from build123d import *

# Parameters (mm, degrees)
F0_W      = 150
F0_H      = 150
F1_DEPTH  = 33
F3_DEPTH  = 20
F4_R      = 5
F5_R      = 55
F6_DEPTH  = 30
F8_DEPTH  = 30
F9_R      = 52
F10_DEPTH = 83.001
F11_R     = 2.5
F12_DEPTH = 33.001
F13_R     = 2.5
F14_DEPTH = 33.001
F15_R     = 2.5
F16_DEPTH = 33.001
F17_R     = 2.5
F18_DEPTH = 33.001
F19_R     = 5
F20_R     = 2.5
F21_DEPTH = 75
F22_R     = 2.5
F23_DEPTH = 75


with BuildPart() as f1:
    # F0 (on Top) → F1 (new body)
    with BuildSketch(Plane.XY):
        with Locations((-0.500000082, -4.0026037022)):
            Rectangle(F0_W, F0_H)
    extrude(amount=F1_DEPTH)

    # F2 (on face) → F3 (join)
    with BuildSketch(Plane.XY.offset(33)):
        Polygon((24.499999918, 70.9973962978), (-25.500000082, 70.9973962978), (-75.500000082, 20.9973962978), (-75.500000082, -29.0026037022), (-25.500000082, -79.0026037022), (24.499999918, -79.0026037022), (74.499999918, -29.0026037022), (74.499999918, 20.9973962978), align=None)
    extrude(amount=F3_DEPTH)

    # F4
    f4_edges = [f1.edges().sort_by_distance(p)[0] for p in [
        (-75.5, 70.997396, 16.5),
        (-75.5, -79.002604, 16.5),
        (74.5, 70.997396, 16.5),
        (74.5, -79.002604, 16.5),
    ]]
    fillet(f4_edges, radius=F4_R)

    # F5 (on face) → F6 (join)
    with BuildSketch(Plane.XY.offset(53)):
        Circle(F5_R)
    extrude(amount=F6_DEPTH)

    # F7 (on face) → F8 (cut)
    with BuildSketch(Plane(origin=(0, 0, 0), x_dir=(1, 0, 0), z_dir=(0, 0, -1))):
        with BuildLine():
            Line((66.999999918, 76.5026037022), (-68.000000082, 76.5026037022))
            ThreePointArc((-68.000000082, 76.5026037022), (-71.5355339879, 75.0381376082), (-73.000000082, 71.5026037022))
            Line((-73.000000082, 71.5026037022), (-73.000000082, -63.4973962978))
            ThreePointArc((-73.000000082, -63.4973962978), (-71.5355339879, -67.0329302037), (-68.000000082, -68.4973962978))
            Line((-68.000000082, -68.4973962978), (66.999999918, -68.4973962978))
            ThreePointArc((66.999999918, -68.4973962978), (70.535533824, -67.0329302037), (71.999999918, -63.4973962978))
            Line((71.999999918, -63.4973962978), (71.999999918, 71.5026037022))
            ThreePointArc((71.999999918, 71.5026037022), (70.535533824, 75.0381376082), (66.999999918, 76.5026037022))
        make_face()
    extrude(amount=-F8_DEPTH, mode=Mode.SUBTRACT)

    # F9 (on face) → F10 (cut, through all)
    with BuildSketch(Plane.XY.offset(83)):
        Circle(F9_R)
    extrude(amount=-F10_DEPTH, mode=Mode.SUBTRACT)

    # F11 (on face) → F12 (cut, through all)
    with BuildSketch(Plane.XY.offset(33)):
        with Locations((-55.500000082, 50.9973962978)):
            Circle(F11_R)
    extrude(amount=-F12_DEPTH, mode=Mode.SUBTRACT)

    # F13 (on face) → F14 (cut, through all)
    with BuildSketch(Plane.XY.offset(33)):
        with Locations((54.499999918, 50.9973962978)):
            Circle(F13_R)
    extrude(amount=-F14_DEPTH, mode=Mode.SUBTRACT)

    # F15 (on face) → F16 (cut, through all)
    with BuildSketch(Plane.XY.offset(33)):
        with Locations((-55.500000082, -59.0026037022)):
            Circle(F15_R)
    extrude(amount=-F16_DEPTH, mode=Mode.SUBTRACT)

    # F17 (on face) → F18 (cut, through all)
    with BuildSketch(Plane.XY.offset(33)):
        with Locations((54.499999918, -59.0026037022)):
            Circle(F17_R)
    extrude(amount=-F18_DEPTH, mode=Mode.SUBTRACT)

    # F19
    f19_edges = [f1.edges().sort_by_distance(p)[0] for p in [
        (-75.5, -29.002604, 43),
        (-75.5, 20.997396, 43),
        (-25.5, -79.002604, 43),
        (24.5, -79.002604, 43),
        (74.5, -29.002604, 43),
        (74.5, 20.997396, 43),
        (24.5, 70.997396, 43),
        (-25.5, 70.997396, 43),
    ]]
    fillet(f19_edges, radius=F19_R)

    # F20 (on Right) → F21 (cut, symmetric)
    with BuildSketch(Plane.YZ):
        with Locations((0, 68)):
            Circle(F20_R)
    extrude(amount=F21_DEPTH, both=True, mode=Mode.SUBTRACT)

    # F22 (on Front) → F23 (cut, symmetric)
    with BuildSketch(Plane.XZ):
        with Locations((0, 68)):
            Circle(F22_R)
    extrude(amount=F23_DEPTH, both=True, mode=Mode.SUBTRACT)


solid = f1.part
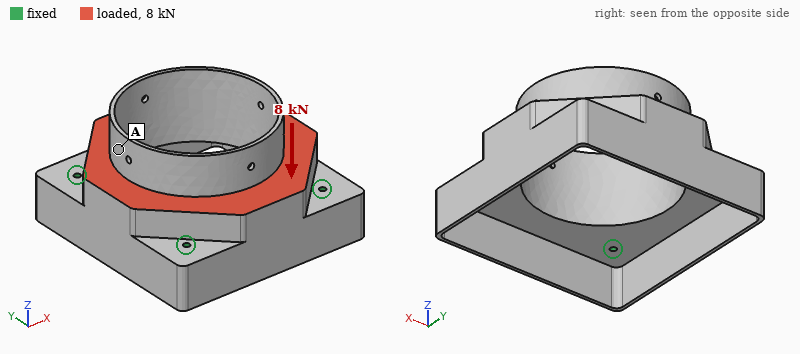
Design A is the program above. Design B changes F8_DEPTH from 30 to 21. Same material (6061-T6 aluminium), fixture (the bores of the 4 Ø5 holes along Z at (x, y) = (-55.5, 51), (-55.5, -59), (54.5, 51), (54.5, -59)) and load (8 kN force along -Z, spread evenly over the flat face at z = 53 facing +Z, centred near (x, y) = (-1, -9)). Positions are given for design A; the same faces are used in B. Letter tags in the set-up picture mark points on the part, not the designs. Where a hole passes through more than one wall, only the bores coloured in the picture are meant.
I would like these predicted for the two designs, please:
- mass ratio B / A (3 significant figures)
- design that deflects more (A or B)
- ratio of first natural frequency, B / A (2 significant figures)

1.38
A
1.8
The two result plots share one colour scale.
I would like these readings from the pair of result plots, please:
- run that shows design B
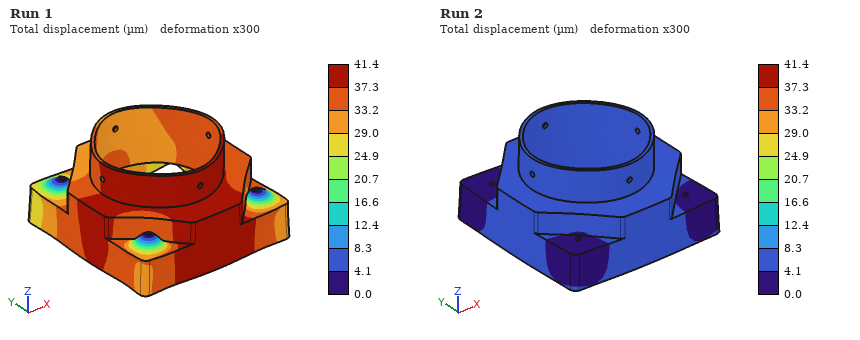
Run 2
